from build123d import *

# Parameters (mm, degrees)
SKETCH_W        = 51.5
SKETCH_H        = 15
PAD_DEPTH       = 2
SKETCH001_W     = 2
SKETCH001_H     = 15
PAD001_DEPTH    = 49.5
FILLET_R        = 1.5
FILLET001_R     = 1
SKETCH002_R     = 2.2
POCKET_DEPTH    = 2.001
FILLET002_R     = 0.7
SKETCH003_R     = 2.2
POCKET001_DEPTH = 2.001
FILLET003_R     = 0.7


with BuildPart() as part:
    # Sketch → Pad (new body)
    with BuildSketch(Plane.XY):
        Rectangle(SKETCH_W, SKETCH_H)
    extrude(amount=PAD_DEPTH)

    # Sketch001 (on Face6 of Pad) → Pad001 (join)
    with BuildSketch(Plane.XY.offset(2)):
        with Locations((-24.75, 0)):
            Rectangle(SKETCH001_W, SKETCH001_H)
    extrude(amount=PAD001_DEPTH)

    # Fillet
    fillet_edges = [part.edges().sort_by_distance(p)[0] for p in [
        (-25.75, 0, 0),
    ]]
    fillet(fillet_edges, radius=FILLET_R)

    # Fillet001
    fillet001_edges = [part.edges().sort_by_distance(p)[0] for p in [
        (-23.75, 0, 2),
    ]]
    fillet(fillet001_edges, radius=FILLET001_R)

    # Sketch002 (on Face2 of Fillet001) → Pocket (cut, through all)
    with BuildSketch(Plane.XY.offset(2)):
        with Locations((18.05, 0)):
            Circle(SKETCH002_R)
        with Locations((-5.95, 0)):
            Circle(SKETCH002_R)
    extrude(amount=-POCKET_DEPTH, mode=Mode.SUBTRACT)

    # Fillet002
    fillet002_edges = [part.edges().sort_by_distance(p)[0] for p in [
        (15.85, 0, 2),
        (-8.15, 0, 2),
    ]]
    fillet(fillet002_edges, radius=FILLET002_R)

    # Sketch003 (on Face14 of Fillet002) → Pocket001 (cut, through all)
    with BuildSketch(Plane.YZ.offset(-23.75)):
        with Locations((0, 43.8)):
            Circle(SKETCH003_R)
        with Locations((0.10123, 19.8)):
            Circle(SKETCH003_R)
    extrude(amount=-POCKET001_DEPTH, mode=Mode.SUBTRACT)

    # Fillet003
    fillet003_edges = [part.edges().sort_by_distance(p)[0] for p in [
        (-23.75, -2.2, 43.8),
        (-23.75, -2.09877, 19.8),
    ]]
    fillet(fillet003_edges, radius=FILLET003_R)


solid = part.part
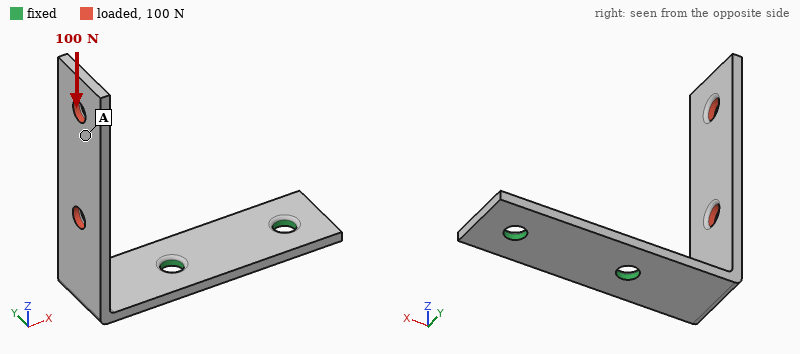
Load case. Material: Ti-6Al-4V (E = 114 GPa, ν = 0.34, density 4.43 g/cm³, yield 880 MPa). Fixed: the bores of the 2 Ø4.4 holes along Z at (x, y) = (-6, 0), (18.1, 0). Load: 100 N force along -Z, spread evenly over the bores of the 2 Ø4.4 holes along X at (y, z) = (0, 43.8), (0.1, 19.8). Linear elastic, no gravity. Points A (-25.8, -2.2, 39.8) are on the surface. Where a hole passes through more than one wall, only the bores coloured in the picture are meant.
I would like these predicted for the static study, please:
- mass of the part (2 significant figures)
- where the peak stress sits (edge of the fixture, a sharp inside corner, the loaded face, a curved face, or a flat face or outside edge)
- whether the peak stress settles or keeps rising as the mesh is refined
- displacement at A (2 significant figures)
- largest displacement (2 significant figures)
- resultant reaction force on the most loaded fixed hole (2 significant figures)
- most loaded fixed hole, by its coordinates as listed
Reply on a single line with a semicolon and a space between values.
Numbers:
13 g; edge of the fixture; keeps rising; 0.63 mm; 0.80 mm; 110 N; (-6, 0)
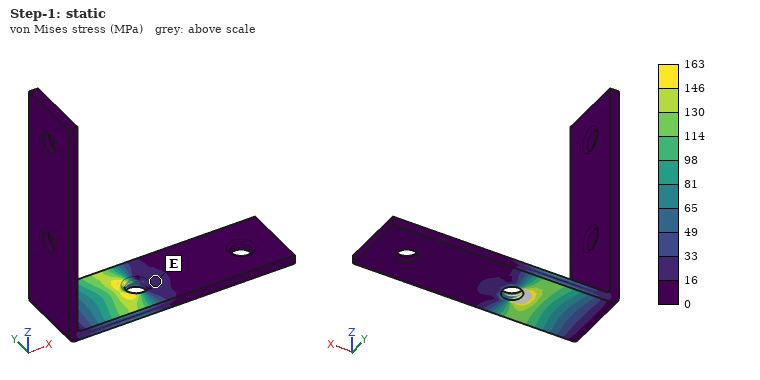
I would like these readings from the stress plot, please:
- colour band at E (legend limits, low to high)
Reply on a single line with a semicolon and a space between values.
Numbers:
16 to 33 MPa
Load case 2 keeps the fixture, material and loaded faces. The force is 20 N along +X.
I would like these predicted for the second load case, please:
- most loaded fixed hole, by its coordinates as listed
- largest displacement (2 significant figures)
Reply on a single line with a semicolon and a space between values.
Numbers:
(18.1, 0); 0.82 mm
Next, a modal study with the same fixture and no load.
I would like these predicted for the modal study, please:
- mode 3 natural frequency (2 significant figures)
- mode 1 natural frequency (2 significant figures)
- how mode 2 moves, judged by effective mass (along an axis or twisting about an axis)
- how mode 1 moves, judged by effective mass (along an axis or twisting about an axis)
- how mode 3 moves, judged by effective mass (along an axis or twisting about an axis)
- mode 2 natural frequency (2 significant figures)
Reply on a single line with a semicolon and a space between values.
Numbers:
1800 Hz; 420 Hz; along Y; along X; along Z; 680 Hz
